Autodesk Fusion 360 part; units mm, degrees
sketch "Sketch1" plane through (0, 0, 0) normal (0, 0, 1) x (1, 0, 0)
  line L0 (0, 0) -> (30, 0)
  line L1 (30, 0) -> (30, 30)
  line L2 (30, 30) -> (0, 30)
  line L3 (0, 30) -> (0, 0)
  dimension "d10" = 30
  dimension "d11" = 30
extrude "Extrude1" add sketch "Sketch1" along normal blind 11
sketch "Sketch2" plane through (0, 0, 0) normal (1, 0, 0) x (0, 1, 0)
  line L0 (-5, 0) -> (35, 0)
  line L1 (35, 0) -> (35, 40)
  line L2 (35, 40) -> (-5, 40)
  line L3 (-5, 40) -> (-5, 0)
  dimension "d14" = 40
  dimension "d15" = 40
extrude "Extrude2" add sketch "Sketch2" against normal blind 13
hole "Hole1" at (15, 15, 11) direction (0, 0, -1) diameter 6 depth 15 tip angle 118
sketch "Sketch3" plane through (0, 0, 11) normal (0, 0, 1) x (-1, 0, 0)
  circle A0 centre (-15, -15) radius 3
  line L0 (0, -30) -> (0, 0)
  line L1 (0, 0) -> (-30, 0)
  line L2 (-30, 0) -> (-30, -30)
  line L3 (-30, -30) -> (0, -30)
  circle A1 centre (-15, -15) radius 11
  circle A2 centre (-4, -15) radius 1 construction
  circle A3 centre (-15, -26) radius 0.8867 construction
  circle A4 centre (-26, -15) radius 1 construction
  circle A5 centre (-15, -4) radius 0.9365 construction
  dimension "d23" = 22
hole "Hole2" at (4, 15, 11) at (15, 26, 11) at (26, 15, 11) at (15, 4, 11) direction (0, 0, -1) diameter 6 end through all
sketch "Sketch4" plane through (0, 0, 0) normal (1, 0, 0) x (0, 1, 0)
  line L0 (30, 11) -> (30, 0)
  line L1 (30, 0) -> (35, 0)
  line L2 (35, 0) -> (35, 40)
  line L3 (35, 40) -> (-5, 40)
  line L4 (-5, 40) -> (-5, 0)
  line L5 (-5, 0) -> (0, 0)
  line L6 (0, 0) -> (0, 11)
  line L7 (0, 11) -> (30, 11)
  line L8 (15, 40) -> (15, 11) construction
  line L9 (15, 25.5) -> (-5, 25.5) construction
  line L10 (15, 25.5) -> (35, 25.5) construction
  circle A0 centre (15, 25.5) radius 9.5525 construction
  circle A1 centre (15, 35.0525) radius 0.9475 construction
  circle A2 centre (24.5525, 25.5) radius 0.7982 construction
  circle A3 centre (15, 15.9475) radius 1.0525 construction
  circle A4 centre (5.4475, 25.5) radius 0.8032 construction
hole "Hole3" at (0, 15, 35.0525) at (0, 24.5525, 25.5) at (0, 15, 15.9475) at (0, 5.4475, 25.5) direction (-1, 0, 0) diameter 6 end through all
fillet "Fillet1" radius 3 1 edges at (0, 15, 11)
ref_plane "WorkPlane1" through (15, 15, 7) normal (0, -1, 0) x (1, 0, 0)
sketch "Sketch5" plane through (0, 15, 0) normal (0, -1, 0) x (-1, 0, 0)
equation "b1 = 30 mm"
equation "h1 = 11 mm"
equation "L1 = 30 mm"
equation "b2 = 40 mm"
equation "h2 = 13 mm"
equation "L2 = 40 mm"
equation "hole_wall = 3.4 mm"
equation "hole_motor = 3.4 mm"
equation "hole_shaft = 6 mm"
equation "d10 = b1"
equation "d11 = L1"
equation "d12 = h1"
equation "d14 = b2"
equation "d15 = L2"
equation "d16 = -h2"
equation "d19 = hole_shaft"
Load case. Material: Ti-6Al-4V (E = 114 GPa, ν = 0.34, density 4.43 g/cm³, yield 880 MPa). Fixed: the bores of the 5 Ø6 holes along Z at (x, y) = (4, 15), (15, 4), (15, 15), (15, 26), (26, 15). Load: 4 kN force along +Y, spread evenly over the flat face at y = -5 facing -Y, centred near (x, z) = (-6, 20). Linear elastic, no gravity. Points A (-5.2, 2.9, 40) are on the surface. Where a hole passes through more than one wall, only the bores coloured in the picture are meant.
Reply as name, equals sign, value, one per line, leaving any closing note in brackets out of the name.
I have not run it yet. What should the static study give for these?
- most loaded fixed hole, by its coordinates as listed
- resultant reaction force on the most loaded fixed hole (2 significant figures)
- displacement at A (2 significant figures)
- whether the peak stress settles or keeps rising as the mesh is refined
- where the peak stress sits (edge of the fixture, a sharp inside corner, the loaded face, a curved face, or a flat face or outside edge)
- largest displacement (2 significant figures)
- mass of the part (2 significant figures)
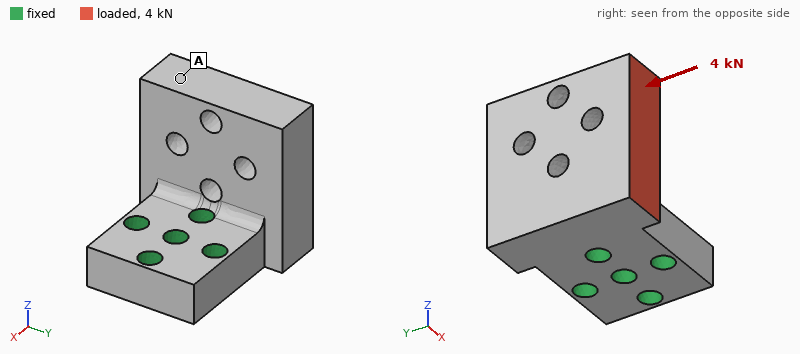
most loaded fixed hole, by its coordinates as listed = (4, 15)
resultant reaction force on the most loaded fixed hole = 4.2 kN
displacement at A = 37 µm
whether the peak stress settles or keeps rising as the mesh is refined = keeps rising
where the peak stress sits = edge of the fixture
largest displacement = 40 µm
mass of the part = 120 g
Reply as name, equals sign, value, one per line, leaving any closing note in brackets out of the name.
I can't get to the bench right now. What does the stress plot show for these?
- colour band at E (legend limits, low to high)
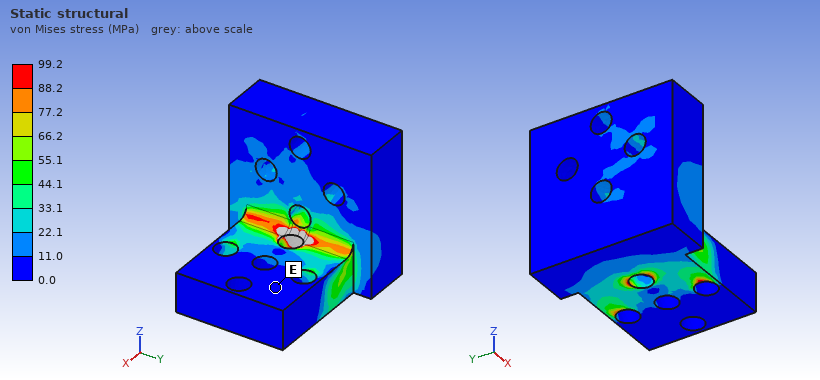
colour band at E = 0.0 to 11.0 MPa
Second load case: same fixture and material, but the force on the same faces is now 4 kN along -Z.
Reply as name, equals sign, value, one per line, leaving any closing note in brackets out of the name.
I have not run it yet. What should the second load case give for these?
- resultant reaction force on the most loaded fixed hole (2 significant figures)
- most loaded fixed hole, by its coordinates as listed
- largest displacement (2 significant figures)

resultant reaction force on the most loaded fixed hole = 4.0 kN
most loaded fixed hole, by its coordinates as listed = (4, 15)
largest displacement = 67 µm
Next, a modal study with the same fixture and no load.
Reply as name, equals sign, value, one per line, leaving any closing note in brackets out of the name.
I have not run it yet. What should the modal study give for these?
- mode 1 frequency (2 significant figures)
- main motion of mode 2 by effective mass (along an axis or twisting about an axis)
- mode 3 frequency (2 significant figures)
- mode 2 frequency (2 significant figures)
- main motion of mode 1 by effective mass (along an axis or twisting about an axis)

mode 1 frequency = 5200 Hz
main motion of mode 2 by effective mass = along Y
mode 3 frequency = 11 kHz
mode 2 frequency = 6200 Hz
main motion of mode 1 by effective mass = along X
